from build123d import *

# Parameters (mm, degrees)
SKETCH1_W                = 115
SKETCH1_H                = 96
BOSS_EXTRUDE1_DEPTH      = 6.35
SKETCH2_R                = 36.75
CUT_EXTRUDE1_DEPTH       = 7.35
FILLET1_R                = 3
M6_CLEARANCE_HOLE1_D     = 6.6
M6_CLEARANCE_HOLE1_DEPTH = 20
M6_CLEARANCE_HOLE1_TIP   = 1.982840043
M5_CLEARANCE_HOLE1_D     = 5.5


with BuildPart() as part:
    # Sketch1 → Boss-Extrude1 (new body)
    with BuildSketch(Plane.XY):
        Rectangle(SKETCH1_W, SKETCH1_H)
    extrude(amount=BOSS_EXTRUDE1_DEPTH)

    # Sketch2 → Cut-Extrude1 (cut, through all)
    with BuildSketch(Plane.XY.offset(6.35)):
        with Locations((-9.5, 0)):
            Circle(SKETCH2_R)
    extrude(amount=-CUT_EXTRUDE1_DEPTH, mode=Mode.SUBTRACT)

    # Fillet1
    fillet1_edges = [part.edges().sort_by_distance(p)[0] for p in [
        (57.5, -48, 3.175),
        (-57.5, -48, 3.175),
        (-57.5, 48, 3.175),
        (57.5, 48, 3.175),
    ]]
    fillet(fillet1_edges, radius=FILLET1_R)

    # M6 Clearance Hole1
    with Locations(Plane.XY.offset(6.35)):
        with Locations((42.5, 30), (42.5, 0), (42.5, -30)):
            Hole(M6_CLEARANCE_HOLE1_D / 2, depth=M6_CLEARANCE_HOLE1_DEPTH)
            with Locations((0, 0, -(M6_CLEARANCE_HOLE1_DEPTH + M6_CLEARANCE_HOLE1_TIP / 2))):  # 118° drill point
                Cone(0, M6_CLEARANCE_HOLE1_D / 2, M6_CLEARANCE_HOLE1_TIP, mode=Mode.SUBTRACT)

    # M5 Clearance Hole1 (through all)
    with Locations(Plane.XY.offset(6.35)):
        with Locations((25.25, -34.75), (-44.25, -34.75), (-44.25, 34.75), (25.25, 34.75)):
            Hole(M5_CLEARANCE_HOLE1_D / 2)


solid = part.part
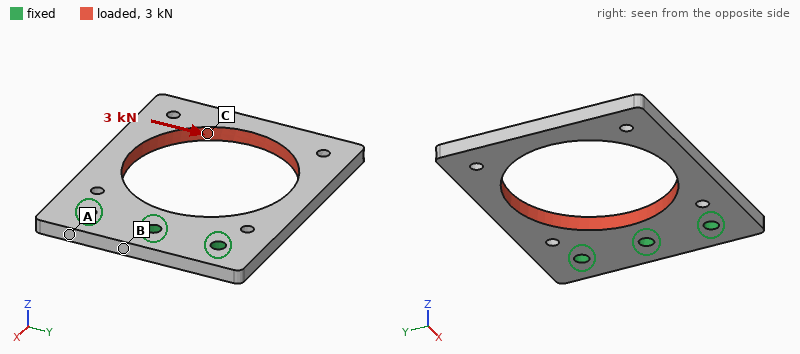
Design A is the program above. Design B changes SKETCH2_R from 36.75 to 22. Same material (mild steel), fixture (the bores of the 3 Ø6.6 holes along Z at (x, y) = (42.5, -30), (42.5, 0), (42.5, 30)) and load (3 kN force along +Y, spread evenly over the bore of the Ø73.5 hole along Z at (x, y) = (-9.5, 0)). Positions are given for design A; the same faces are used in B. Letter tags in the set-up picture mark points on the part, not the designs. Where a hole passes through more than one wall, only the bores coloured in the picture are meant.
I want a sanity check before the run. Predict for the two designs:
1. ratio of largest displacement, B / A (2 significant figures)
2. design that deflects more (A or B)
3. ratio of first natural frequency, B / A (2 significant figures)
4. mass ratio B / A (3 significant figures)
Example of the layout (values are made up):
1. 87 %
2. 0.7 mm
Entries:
1. 0.24
2. A
3. 1.2
4. 1.41
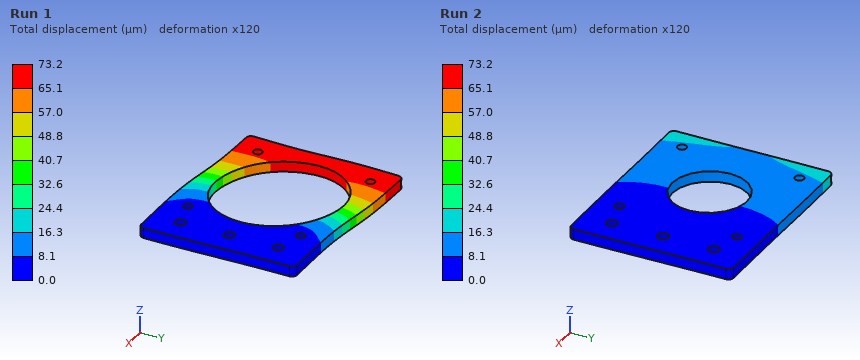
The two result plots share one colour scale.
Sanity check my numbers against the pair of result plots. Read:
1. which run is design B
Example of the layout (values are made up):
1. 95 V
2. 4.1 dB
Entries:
1. Run 2
